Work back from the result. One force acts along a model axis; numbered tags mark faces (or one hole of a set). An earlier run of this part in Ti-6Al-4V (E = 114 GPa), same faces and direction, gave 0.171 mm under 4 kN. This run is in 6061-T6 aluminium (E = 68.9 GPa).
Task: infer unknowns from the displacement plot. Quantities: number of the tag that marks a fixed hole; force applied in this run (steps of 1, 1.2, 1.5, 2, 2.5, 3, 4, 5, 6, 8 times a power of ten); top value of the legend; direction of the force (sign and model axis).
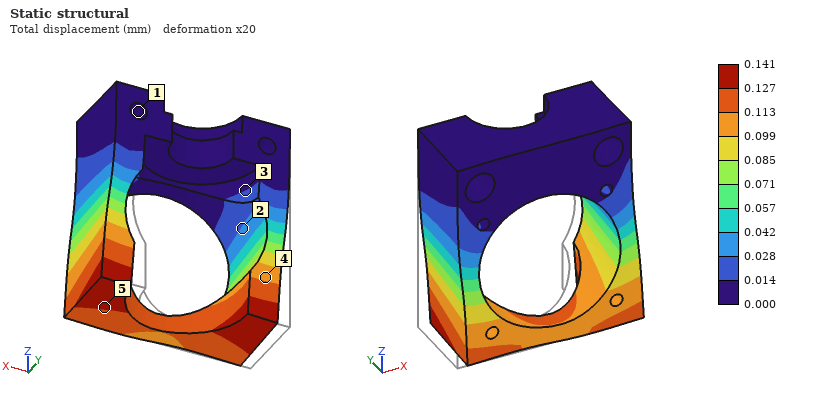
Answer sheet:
1
2 kN
0.141 mm
+X
